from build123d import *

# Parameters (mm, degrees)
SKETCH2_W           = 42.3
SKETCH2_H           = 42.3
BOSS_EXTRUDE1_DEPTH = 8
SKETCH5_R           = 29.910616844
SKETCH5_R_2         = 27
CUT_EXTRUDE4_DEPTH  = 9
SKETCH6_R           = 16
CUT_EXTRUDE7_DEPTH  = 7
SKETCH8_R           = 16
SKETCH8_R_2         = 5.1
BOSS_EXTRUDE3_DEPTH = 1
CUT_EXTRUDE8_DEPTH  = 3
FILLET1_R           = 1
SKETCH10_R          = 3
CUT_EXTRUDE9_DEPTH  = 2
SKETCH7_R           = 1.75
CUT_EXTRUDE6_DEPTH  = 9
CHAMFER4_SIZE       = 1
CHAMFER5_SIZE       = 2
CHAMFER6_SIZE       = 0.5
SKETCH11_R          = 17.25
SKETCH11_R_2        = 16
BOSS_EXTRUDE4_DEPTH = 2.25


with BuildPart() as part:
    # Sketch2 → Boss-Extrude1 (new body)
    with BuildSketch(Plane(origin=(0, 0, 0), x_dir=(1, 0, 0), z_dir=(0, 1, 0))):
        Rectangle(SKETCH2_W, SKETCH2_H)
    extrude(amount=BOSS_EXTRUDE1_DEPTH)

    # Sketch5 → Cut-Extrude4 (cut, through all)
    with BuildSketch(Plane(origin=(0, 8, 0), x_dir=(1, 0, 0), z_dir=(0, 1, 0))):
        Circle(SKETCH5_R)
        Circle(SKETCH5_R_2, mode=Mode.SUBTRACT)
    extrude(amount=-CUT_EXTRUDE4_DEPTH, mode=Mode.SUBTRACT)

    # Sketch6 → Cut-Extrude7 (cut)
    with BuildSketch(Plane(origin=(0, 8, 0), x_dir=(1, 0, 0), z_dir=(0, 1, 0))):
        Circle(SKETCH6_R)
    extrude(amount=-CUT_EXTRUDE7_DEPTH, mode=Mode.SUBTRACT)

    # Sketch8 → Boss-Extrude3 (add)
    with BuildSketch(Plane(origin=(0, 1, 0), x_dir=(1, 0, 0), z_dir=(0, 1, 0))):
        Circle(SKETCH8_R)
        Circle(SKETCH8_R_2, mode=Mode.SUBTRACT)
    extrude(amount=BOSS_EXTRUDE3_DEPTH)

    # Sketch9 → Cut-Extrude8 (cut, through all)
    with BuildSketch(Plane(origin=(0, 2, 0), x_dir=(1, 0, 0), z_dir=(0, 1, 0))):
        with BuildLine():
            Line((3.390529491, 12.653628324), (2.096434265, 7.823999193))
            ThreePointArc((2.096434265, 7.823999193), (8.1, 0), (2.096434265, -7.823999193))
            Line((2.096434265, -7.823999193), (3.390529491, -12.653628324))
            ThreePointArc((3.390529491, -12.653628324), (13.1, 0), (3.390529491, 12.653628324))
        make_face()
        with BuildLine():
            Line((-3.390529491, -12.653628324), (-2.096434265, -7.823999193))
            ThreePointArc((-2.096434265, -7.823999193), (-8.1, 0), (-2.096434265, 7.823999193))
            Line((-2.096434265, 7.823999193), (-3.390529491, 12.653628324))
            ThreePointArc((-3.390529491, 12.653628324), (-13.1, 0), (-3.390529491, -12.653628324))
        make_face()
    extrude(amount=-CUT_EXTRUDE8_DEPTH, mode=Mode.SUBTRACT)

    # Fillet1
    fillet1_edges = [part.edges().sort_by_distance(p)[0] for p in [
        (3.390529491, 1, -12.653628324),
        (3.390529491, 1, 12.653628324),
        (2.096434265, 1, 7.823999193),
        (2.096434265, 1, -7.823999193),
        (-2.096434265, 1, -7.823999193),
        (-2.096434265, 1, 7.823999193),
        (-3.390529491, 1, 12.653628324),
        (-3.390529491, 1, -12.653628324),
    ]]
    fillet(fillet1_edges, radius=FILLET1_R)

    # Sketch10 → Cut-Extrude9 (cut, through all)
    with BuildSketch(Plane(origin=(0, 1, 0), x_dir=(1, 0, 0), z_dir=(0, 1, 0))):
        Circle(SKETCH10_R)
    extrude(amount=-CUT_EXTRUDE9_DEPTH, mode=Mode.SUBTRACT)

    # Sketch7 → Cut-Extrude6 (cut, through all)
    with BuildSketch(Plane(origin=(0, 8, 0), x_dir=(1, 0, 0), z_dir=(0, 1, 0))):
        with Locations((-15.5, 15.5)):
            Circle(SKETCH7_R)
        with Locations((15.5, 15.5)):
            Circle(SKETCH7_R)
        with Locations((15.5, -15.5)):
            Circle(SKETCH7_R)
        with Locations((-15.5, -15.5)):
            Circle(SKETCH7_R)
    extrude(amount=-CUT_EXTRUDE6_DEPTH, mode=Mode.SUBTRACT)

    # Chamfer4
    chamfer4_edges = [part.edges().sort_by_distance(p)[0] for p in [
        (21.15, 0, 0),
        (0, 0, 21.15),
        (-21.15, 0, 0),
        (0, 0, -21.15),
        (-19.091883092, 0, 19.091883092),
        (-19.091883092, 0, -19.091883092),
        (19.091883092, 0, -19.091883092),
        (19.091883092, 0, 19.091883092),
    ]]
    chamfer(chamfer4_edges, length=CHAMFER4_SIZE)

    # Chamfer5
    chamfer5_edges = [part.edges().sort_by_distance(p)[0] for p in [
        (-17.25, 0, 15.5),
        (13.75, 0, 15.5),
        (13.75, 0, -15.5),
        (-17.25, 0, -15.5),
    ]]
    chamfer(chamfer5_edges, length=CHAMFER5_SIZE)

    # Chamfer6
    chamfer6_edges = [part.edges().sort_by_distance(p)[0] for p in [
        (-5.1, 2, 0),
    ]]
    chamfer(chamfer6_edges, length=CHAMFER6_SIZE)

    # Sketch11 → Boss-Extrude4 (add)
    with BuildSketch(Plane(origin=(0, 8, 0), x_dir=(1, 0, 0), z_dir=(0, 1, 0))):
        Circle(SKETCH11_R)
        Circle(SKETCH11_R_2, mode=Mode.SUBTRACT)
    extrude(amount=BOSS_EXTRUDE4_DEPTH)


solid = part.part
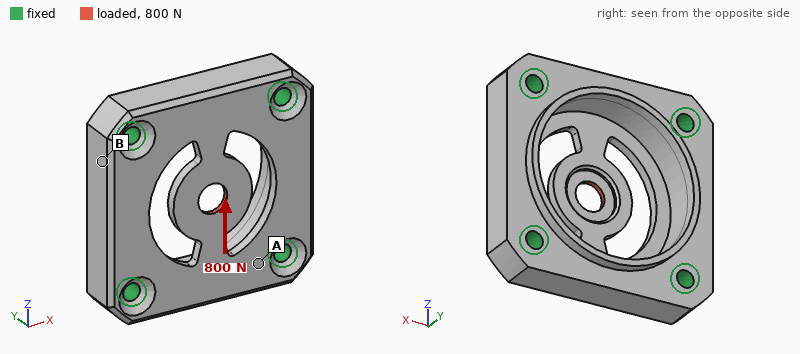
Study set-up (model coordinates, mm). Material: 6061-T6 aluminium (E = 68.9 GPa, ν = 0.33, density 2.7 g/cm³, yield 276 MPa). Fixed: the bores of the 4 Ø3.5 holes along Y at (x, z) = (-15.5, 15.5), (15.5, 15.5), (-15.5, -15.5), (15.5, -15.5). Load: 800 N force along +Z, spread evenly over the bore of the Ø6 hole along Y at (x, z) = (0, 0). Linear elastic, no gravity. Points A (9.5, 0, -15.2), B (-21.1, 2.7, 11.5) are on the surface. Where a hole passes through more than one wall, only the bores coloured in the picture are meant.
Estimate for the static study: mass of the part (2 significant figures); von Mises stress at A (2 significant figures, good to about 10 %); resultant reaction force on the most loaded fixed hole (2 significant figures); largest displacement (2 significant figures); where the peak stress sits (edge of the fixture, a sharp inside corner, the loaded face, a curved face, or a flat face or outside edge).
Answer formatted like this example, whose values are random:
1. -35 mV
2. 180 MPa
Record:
1. 22 g
2. 13 MPa
3. 210 N
4. 14 µm
5. a curved face
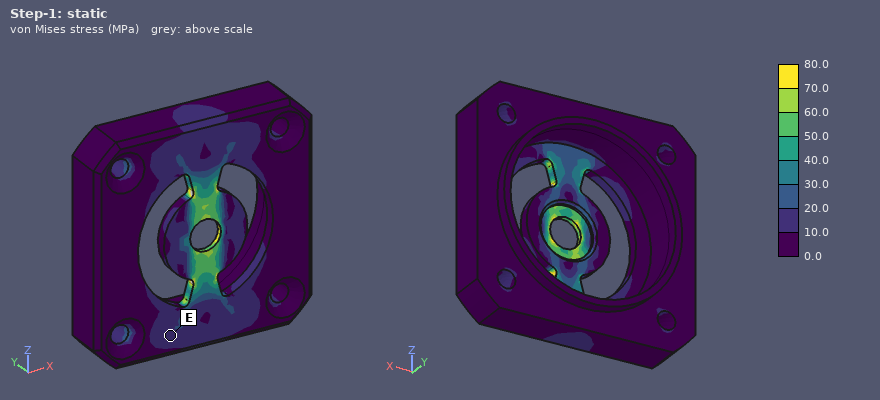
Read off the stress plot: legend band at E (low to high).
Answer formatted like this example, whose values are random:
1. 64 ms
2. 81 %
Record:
1. 10.0 to 20.0 MPa
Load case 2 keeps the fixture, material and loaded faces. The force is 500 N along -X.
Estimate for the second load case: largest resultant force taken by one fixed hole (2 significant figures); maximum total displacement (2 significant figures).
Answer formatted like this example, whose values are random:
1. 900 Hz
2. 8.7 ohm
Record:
1. 150 N
2. 35 µm
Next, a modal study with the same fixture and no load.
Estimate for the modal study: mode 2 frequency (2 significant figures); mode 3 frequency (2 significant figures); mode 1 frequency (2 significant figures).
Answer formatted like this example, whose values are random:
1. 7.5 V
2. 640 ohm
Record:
1. 10 kHz
2. 21 kHz
3. 8400 Hz
